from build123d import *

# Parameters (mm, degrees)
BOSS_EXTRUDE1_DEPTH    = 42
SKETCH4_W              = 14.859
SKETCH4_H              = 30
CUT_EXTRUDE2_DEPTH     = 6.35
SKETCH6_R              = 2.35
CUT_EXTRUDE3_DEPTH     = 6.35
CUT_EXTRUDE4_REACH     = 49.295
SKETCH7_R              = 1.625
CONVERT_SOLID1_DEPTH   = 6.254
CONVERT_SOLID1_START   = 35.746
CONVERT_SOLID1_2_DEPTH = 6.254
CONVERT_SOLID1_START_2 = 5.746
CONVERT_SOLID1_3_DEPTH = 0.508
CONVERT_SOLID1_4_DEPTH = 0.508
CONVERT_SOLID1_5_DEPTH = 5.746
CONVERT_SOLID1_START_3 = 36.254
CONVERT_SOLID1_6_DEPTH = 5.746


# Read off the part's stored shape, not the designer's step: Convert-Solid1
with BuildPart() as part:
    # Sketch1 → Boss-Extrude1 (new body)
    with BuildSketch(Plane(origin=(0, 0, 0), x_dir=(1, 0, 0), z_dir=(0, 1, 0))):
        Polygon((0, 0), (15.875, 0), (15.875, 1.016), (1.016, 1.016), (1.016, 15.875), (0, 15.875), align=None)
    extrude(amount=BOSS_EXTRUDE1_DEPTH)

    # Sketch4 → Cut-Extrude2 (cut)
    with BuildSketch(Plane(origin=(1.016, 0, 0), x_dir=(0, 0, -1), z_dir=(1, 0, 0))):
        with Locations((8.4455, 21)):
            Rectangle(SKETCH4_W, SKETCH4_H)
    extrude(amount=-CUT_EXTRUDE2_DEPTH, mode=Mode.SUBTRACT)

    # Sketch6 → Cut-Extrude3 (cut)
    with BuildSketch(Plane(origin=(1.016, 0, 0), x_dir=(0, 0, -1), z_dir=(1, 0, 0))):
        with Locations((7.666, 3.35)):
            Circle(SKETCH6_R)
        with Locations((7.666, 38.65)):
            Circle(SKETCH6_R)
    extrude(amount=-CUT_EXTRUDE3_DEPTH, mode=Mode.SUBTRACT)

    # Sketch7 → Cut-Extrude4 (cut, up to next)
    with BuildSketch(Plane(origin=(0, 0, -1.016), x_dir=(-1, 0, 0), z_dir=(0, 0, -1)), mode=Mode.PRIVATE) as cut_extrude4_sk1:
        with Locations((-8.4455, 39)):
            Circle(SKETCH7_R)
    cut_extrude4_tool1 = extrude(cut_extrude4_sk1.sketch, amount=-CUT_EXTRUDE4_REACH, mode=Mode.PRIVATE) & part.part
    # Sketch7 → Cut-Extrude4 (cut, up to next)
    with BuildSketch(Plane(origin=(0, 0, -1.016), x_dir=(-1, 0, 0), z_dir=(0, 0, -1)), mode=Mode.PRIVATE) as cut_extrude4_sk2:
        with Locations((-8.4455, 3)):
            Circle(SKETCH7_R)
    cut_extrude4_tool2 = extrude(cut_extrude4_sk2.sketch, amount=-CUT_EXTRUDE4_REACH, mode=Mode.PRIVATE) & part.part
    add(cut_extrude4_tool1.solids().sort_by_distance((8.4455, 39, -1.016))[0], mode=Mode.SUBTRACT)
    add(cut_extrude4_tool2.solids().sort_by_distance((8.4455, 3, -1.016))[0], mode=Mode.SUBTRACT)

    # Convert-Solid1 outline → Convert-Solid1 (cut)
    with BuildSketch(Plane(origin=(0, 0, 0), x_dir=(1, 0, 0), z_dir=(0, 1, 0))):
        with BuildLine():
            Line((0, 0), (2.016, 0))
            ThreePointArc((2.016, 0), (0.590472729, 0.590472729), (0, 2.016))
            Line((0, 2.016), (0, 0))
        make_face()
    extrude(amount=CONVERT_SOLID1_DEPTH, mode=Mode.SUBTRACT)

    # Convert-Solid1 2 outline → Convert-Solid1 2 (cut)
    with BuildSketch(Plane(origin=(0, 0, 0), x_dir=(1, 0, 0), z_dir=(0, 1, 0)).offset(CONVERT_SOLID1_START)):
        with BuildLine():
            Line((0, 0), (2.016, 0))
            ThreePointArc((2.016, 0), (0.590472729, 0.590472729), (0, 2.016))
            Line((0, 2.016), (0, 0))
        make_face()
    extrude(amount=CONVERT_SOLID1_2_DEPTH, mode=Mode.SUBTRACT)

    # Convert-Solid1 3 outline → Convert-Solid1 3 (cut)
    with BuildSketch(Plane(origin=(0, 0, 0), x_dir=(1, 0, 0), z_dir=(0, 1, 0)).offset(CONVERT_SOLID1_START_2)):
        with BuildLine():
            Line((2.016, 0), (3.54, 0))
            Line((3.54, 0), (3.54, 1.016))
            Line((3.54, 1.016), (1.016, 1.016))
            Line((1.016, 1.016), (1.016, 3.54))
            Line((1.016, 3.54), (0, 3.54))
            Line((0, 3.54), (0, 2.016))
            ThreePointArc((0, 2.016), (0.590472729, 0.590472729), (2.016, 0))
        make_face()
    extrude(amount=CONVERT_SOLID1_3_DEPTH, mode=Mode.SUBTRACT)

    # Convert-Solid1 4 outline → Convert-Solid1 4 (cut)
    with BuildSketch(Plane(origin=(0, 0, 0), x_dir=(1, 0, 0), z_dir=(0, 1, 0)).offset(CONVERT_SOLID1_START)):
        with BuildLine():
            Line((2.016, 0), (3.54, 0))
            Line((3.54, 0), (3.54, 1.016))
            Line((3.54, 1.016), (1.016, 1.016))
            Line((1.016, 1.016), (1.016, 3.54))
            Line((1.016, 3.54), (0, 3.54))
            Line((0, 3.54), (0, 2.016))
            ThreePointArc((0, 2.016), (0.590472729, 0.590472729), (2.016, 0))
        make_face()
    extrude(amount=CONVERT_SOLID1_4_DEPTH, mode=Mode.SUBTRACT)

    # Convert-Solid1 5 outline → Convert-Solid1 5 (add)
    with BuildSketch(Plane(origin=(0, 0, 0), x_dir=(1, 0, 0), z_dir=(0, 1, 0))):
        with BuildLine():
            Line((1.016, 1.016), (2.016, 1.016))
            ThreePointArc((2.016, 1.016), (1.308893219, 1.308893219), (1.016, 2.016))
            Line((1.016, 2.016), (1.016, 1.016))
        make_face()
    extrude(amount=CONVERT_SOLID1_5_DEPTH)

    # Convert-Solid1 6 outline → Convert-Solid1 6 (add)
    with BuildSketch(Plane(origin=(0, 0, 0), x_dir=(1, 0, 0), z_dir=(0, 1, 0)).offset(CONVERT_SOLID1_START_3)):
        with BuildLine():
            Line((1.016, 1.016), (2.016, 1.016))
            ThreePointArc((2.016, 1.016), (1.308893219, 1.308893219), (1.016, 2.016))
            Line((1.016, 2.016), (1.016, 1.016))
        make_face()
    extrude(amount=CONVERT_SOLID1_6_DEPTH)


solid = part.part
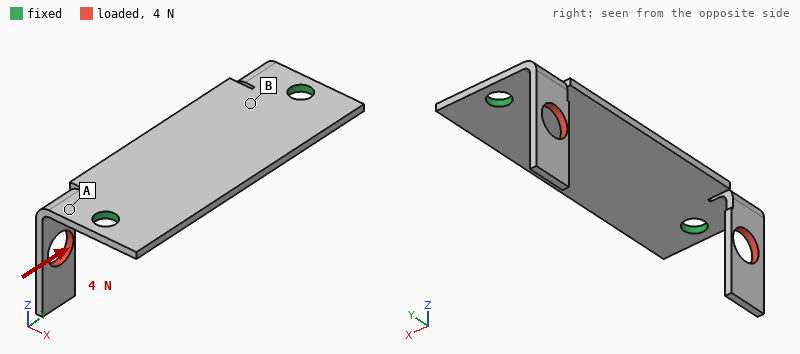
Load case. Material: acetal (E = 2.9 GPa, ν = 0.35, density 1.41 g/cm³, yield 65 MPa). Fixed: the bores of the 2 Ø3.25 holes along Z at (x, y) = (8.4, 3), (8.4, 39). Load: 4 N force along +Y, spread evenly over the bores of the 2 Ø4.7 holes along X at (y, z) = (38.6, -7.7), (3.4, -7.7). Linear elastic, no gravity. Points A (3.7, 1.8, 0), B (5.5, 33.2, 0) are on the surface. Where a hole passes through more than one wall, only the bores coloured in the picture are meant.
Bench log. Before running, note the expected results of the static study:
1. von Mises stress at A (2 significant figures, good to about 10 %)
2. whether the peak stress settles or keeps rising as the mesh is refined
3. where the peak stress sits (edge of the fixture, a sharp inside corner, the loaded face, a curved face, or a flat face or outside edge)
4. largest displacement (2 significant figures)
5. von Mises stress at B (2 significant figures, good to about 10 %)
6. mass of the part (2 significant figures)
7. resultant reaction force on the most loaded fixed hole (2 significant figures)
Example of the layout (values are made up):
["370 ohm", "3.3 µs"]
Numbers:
["9.5 MPa", "keeps rising", "a sharp inside corner", "0.54 mm", "1.8 MPa", "1.1 g", "2.1 N"]
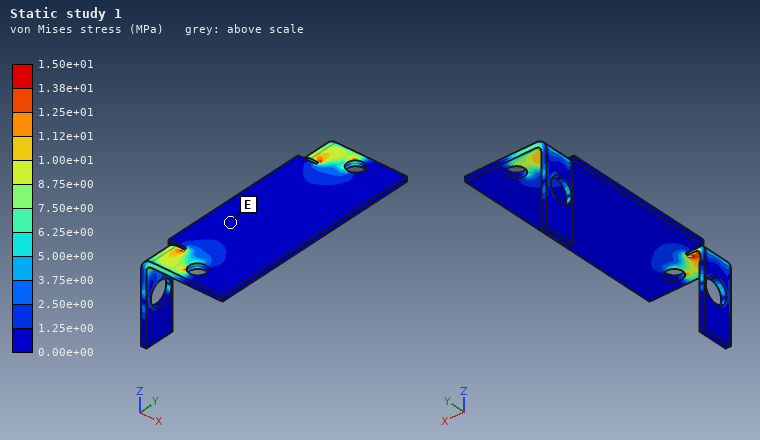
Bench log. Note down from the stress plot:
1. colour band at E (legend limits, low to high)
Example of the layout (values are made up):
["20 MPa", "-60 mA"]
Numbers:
["0.00e+00 to 1.25e+00 MPa"]
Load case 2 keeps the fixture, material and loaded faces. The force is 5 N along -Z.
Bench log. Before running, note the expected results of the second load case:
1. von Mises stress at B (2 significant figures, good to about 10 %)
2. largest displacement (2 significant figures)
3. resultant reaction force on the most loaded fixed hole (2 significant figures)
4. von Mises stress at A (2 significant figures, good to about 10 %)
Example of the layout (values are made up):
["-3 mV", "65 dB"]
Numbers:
["1.9 MPa", "0.49 mm", "2.5 N", "6.3 MPa"]
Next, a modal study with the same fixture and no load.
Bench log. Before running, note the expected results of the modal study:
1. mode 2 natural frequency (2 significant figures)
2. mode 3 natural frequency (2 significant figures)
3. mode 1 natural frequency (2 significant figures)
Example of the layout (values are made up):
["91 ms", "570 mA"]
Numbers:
["600 Hz", "990 Hz", "600 Hz"]
